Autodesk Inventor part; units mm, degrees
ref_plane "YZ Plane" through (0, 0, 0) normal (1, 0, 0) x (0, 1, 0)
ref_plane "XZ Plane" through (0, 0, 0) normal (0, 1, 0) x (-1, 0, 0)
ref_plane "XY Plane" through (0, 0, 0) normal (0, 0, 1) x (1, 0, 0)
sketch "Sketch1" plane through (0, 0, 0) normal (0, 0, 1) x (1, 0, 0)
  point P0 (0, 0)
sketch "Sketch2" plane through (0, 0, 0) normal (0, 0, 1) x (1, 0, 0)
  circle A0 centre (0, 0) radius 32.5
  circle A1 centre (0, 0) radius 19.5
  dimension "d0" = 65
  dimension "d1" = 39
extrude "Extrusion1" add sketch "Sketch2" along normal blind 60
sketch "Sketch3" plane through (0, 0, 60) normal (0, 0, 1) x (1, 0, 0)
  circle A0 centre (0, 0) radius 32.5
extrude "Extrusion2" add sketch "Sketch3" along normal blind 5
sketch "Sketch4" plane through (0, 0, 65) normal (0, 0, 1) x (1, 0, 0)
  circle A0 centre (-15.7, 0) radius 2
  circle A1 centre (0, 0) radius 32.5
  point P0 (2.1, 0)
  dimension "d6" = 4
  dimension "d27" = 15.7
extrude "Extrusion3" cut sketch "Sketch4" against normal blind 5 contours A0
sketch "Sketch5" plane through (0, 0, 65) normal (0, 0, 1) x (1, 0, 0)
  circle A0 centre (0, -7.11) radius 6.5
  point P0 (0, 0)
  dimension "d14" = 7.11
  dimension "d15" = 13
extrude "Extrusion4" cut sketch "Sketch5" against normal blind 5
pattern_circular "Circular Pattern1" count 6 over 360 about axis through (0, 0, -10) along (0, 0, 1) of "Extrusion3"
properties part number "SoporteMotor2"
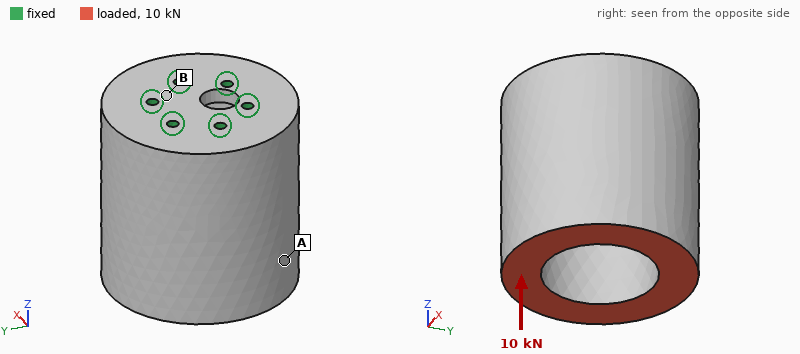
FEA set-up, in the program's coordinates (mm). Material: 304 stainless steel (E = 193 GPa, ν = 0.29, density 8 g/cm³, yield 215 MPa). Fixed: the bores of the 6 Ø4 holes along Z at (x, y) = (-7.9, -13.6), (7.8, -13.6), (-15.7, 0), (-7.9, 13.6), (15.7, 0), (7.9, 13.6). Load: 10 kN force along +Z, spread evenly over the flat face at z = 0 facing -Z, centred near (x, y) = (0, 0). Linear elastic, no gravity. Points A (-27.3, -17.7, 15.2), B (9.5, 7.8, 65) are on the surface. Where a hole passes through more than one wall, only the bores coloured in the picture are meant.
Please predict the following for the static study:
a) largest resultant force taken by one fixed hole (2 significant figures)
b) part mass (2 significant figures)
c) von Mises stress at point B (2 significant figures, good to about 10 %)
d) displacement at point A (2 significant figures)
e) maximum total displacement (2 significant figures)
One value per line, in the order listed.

1.7 kN
1.1 kg
16 MPa
4.2 µm
4.7 µm
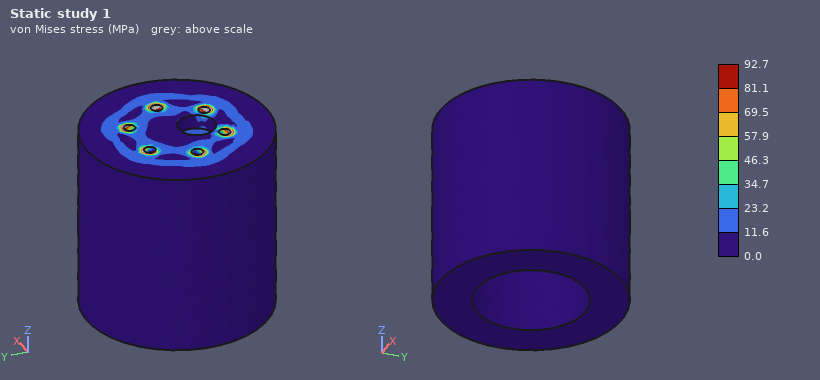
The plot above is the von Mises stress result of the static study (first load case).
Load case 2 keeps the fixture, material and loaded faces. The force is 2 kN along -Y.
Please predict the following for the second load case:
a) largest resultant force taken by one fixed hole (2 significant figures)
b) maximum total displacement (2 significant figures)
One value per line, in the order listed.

1.9 kN
20 µm
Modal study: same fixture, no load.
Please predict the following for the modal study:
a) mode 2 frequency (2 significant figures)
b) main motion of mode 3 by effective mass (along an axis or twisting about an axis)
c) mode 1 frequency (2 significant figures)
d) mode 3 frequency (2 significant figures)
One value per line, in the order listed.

2500 Hz
twisting about Z
2500 Hz
7300 Hz
